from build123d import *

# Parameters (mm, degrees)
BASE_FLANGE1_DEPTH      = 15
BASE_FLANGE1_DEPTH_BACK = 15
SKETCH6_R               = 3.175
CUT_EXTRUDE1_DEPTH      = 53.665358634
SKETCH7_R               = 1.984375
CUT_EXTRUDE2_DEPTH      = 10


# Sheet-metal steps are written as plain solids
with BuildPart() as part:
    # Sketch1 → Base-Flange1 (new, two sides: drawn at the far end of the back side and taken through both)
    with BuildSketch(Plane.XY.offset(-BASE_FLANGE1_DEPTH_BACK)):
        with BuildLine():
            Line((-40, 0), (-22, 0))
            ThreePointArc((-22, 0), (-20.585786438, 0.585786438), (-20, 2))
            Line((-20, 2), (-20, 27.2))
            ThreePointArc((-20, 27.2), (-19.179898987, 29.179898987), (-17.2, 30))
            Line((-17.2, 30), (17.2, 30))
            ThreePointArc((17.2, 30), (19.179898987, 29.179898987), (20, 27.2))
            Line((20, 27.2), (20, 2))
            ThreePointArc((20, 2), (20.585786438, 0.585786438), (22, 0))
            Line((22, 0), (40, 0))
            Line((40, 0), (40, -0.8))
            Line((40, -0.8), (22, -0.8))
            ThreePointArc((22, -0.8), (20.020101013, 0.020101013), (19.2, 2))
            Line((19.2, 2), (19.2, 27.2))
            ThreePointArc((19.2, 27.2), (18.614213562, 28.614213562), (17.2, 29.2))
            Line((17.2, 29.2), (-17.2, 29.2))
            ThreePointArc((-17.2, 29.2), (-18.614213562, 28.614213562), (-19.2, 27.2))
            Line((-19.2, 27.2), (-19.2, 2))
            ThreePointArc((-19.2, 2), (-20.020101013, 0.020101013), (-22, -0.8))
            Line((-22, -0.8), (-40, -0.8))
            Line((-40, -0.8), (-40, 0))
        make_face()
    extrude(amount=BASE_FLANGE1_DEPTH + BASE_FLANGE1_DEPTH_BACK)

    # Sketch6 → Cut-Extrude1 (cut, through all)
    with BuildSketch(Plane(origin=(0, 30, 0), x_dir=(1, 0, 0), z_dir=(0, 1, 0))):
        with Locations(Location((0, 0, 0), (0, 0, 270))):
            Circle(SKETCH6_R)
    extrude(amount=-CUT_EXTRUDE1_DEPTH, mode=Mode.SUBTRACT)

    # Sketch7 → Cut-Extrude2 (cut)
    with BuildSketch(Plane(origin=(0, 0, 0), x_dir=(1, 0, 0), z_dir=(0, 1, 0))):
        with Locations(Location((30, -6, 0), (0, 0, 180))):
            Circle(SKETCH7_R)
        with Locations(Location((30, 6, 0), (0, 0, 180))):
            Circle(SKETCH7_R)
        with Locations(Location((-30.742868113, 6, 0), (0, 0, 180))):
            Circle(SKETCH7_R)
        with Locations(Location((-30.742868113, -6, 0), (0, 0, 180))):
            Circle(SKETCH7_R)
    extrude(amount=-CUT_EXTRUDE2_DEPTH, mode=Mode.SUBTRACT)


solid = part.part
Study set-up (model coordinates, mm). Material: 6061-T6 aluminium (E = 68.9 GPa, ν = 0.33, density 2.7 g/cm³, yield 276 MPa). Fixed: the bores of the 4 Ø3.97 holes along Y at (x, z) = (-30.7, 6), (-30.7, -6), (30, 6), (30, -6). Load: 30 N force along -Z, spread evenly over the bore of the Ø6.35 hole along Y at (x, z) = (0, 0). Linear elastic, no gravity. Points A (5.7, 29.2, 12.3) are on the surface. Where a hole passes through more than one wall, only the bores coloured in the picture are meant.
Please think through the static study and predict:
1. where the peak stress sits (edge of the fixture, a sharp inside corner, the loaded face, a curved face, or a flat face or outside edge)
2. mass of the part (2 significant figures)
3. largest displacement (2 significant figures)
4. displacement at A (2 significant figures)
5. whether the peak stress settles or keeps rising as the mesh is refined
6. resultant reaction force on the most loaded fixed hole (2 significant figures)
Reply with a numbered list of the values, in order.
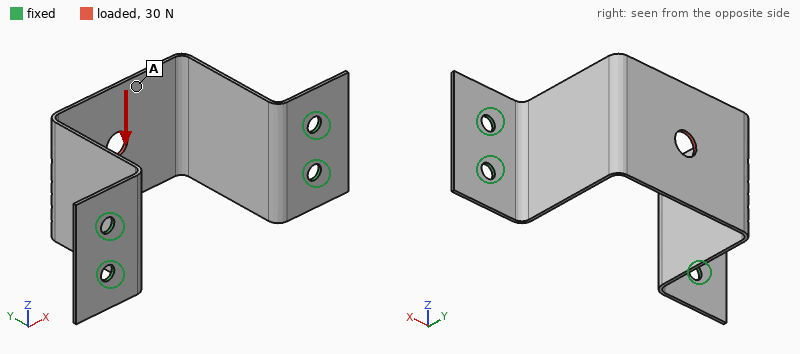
1. edge of the fixture
2. 8.6 g
3. 0.34 mm
4. 0.30 mm
5. keeps rising
6. 32 N
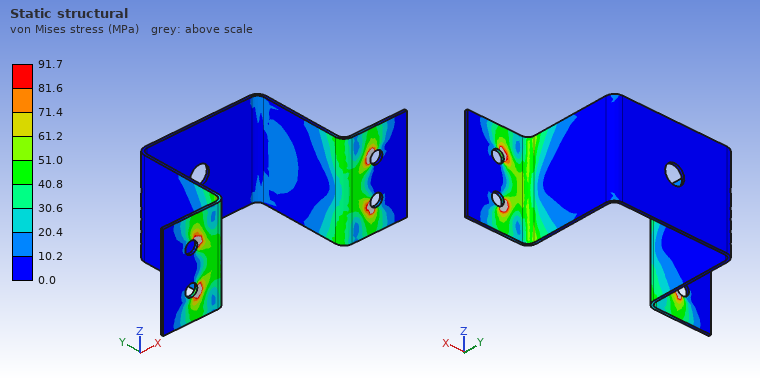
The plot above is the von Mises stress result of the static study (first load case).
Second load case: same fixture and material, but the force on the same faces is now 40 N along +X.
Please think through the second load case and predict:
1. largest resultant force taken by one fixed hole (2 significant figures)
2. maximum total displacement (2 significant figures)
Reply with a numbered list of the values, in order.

1. 13 N
2. 0.94 mm
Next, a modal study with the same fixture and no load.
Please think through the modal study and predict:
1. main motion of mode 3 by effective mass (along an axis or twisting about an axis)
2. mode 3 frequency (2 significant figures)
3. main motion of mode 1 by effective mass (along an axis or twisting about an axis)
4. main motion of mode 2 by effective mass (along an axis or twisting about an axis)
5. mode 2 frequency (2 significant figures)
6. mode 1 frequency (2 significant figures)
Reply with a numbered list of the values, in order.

1. twisting about Y
2. 990 Hz
3. along X
4. along Z
5. 790 Hz
6. 530 Hz
